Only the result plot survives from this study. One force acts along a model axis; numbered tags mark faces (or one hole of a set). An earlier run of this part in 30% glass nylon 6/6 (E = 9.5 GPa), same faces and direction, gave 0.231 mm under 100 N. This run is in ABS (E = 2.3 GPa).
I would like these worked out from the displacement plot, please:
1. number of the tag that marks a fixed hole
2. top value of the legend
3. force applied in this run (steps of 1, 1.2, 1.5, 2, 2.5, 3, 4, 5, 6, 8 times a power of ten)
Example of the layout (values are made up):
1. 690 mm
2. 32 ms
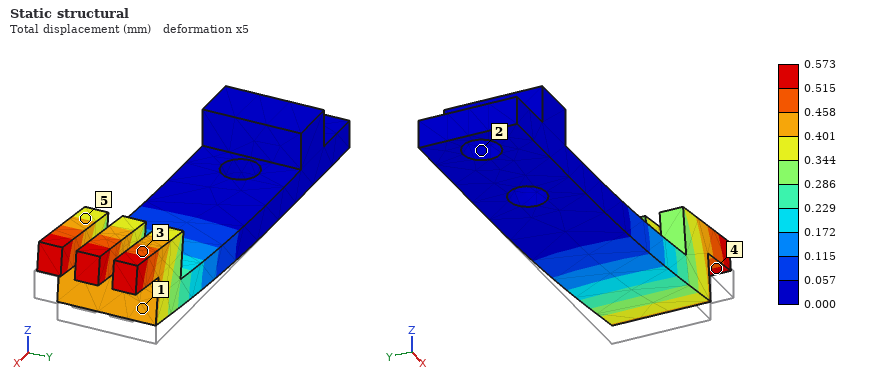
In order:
1. 2
2. 0.573 mm
3. 60 N
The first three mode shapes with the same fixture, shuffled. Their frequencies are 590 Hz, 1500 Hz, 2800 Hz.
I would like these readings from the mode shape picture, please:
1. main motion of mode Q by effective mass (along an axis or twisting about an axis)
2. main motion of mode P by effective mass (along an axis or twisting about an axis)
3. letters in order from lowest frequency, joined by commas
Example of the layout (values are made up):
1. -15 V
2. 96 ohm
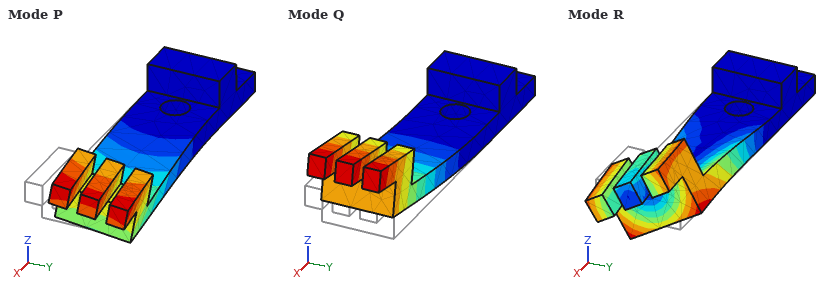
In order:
1. along Z
2. along Y
3. Q, P, R
